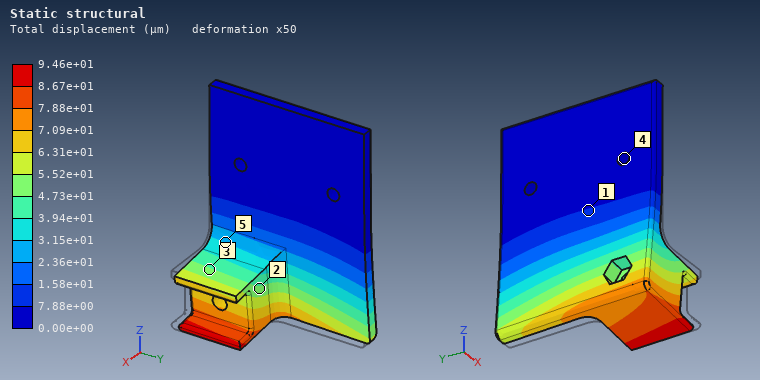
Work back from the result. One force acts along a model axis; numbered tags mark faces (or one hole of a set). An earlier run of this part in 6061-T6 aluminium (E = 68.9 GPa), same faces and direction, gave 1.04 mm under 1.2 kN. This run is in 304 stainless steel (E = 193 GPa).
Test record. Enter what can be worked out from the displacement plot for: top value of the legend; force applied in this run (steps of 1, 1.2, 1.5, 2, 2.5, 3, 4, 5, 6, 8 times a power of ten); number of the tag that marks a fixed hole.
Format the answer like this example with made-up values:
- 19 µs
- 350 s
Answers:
- 9.46e+01 µm
- 300 N
- 4
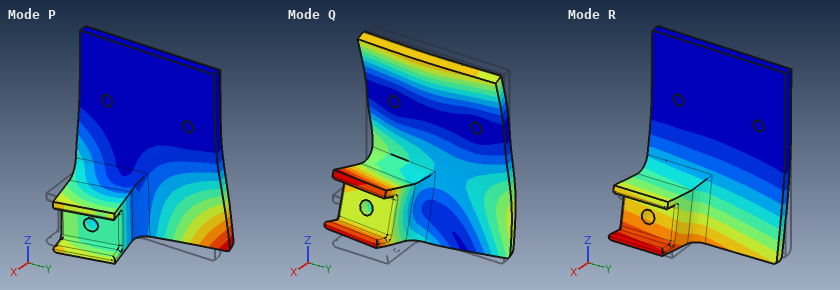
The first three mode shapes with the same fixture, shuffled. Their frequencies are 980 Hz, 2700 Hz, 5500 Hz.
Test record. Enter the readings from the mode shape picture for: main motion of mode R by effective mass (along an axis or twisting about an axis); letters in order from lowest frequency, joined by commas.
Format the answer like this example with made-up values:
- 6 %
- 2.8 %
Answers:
- along X
- R, P, Q
